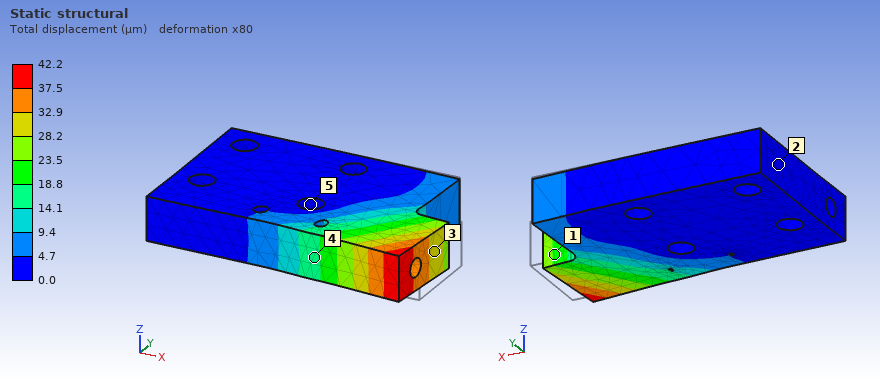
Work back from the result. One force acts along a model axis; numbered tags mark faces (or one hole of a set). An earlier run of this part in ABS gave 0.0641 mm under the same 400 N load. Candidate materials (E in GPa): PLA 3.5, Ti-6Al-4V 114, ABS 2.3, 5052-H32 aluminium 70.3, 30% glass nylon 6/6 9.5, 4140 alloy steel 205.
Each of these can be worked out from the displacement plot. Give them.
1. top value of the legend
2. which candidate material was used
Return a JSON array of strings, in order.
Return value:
["42.2 µm", "PLA"]
